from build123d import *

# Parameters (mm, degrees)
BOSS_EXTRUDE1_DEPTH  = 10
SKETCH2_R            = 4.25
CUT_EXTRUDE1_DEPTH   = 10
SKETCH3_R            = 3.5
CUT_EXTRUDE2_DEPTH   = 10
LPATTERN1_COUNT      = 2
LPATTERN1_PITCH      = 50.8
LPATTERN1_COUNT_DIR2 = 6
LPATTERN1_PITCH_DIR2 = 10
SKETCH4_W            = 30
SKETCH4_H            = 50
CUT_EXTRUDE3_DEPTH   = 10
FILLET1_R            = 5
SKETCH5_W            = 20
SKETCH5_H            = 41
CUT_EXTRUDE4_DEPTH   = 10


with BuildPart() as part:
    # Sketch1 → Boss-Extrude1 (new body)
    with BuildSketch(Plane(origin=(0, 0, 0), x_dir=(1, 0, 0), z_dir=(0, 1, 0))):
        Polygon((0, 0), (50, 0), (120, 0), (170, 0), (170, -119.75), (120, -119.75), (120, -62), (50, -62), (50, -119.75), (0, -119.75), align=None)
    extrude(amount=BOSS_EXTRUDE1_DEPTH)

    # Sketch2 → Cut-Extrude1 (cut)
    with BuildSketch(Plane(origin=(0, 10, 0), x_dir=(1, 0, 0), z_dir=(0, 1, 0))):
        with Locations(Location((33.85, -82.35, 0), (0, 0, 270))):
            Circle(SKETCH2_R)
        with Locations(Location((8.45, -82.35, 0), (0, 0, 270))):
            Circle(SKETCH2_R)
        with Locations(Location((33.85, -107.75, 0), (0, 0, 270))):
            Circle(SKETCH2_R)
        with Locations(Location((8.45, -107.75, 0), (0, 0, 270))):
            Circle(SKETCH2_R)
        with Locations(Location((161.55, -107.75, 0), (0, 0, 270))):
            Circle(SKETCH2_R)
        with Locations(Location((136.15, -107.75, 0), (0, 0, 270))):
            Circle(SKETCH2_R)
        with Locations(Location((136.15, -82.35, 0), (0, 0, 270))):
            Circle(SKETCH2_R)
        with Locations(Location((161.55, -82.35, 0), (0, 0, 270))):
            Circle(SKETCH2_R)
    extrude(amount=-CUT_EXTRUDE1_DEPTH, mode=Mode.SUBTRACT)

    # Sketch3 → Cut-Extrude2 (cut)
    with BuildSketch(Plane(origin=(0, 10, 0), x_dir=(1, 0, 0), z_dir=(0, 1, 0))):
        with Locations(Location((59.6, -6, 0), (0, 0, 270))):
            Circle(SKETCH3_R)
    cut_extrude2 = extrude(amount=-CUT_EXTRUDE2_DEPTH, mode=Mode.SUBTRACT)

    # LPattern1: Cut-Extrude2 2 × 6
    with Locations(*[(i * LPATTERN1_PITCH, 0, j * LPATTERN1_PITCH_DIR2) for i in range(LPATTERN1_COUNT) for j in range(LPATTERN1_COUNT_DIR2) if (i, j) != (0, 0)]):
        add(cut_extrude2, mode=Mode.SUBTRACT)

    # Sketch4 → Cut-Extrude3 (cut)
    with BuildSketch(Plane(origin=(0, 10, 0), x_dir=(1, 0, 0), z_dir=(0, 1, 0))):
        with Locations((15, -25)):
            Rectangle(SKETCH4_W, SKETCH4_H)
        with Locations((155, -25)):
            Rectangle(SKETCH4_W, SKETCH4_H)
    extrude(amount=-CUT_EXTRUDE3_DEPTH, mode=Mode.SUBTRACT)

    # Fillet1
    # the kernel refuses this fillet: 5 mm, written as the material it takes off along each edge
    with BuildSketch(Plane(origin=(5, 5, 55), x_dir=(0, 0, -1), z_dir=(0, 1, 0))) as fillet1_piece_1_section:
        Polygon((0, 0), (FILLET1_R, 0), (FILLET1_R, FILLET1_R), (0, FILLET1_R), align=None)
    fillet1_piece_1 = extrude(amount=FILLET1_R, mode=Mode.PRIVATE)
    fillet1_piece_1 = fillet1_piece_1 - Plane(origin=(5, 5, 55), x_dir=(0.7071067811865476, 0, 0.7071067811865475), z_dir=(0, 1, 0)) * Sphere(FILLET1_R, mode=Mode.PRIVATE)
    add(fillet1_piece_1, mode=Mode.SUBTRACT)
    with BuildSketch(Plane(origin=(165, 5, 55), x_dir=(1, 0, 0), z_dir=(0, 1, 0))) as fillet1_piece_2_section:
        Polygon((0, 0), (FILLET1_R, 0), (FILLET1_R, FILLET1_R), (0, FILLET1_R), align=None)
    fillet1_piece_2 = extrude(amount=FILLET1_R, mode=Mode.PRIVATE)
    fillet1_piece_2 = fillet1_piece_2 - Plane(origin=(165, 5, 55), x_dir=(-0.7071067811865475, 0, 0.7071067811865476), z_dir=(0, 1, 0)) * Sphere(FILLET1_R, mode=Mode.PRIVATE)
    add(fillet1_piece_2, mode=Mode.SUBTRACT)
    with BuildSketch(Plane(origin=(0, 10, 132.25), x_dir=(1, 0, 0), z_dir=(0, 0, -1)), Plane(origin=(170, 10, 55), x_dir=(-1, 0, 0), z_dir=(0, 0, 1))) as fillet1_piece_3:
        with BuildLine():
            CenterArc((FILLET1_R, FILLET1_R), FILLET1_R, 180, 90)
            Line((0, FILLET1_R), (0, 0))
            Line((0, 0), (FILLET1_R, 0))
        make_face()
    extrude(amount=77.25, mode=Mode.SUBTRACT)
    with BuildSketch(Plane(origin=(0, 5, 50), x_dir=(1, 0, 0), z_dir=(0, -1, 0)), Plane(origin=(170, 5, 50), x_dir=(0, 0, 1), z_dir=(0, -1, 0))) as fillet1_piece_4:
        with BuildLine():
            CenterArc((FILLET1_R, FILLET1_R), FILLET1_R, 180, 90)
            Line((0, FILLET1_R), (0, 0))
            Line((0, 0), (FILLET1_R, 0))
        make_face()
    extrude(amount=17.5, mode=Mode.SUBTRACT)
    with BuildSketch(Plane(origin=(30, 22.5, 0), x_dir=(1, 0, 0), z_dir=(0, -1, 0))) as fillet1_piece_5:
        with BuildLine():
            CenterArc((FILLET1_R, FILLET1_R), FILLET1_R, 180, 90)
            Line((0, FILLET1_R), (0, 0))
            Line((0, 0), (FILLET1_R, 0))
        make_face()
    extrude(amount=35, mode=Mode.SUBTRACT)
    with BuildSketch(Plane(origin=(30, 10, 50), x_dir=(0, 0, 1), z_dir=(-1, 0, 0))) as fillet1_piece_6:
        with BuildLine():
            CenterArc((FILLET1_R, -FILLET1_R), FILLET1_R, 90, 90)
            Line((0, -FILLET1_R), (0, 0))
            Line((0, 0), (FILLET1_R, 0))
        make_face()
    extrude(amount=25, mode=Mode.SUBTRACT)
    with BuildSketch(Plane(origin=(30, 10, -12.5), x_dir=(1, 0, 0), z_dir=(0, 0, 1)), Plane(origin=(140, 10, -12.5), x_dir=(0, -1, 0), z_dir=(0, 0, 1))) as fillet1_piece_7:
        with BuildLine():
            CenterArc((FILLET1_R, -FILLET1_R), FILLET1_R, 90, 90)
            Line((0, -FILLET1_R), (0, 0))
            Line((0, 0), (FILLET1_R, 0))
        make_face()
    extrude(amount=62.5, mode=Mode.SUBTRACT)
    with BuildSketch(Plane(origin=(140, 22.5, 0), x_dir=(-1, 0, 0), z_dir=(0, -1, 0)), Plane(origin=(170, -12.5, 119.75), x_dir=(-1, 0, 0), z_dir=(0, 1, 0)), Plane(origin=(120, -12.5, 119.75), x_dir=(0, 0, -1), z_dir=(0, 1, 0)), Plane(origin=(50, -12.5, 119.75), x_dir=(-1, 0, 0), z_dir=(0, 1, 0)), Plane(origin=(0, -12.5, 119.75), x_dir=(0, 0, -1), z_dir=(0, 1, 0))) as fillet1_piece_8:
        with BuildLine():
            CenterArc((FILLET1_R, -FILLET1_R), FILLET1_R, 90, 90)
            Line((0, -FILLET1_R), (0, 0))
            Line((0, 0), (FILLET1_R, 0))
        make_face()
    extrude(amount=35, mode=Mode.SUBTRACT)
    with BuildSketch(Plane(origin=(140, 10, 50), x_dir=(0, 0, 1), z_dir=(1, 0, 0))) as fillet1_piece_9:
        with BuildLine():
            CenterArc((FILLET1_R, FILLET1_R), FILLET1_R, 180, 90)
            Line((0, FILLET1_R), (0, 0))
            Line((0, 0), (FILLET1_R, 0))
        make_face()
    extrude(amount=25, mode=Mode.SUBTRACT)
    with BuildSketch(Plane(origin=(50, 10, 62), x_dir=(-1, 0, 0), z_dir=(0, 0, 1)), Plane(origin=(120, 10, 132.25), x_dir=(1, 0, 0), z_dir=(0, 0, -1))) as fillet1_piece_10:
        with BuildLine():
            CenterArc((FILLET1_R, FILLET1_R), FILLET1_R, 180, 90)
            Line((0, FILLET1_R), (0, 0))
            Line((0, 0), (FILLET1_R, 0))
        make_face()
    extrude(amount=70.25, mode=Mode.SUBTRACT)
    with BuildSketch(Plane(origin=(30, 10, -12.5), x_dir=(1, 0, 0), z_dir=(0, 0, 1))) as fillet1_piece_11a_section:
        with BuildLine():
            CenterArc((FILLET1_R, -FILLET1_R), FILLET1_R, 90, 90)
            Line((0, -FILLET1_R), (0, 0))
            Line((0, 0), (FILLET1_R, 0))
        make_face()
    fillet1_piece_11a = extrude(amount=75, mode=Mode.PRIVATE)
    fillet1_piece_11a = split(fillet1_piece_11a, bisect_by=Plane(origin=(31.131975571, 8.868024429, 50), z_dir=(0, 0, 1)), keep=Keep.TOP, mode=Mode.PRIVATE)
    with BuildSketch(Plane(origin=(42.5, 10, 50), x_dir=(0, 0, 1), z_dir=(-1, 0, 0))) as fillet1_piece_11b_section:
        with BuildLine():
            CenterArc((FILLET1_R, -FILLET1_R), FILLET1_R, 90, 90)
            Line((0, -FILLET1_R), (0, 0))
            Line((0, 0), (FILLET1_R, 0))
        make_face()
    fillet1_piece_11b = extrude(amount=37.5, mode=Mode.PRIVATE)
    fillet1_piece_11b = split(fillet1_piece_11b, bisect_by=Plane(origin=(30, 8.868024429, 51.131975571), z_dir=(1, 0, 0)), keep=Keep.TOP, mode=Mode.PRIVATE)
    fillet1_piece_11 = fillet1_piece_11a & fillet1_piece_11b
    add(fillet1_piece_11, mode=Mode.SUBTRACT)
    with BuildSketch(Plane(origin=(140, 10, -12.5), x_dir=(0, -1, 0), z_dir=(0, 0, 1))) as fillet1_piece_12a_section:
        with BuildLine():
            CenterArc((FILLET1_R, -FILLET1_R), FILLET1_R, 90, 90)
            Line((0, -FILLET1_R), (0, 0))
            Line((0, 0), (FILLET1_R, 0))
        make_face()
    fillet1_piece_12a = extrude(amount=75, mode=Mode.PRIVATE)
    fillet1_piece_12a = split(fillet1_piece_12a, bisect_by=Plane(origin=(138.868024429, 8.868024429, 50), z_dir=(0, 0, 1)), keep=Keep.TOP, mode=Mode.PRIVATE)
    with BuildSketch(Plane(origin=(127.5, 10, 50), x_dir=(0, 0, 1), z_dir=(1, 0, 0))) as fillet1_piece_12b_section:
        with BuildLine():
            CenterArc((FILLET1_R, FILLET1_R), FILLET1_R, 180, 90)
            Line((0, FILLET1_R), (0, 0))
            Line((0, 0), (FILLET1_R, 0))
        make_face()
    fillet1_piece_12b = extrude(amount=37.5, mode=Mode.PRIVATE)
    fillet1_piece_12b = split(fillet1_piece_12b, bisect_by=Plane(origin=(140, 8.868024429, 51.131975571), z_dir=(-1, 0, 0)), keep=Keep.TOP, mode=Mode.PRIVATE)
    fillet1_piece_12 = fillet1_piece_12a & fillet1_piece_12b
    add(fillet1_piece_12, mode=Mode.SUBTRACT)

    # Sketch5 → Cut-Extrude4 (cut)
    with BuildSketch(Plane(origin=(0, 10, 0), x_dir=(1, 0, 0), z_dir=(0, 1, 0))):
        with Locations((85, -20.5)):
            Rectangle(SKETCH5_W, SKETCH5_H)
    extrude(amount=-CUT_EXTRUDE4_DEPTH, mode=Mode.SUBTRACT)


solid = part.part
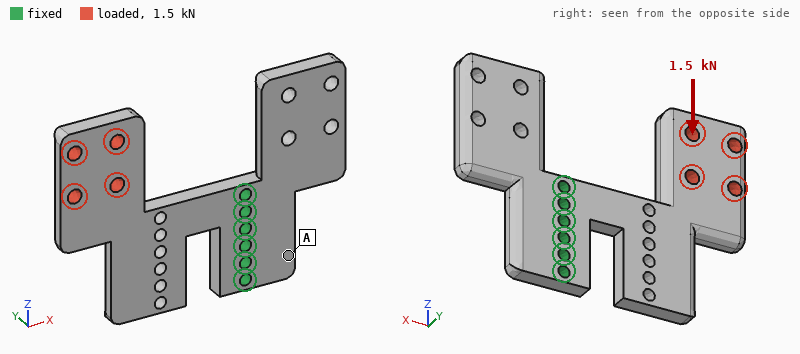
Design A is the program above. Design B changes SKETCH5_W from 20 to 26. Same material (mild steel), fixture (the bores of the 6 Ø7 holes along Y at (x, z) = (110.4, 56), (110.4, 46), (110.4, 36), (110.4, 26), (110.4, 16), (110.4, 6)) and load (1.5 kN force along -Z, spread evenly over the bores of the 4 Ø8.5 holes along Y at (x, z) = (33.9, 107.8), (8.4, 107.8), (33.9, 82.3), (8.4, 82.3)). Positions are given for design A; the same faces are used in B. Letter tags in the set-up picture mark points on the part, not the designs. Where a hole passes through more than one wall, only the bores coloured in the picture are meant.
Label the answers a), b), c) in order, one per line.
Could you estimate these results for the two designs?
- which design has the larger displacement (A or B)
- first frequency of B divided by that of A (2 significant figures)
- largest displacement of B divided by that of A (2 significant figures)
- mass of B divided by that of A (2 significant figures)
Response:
a) B
b) 0.98
c) 1.1
d) 0.98
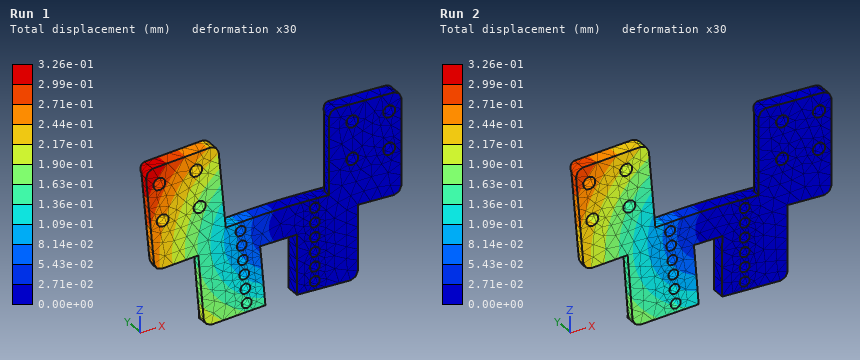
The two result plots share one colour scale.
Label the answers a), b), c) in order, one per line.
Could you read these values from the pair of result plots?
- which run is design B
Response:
a) Run 1
